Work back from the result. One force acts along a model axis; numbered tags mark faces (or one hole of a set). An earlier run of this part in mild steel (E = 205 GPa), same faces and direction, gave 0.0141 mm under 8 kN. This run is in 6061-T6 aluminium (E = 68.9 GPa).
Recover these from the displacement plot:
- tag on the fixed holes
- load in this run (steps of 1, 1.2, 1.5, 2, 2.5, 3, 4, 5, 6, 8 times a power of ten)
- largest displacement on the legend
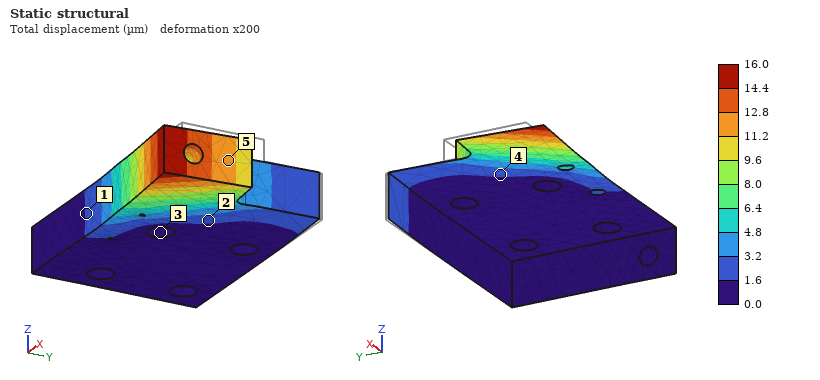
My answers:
3
3 kN
16.0 µm
